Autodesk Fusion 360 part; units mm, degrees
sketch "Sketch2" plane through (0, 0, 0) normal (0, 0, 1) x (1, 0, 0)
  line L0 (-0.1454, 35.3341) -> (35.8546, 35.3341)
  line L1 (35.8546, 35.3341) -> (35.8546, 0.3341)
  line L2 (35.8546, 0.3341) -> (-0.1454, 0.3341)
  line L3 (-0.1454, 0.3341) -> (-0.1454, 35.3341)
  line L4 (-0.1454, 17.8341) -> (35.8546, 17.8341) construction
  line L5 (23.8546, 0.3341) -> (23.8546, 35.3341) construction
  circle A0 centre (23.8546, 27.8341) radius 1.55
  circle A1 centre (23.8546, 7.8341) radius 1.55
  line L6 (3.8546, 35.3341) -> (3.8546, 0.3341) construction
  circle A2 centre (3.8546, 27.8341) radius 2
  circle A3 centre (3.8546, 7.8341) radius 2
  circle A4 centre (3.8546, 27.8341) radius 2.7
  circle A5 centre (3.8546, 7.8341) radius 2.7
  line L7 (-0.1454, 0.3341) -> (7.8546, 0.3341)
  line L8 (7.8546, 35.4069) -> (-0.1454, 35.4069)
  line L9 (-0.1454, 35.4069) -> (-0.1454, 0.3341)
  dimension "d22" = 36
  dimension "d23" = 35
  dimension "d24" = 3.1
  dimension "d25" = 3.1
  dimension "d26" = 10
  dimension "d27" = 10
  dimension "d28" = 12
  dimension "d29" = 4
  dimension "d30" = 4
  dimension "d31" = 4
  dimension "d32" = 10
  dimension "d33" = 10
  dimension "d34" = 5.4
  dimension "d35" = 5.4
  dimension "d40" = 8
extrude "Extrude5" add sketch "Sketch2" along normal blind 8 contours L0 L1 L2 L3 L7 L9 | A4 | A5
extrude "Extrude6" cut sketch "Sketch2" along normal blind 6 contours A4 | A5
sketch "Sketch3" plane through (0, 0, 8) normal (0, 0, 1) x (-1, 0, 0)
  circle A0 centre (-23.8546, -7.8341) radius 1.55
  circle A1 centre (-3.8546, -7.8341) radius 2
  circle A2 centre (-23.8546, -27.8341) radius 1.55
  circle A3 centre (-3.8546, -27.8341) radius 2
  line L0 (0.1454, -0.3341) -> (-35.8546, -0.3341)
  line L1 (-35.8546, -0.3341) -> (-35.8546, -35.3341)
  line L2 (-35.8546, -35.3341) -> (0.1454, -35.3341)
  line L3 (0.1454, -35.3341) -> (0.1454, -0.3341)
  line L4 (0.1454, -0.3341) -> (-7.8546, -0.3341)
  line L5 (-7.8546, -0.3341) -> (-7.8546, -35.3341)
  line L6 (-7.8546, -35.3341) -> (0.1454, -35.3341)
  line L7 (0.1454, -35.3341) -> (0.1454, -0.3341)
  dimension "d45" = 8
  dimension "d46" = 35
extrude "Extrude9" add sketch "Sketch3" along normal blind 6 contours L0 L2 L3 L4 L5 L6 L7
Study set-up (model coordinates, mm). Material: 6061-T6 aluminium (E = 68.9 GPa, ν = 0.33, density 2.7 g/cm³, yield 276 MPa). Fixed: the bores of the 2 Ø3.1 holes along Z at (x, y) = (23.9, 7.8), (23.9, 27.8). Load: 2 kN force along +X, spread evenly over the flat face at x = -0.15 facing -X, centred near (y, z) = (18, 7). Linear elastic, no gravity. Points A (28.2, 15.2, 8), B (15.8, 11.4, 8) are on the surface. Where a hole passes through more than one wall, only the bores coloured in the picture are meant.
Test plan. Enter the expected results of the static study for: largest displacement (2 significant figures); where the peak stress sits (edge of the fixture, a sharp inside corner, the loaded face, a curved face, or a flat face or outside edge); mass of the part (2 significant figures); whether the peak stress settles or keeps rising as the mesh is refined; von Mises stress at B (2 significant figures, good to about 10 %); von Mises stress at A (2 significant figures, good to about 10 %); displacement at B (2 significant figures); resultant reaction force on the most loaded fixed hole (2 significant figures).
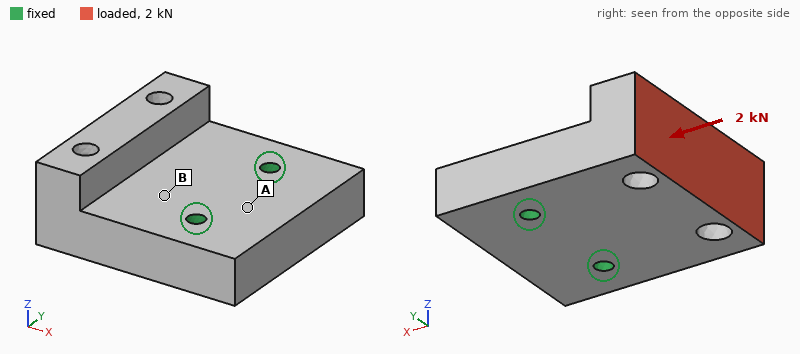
25 µm
edge of the fixture
30 g
keeps rising
22 MPa
5.3 MPa
4.6 µm
1.0 kN
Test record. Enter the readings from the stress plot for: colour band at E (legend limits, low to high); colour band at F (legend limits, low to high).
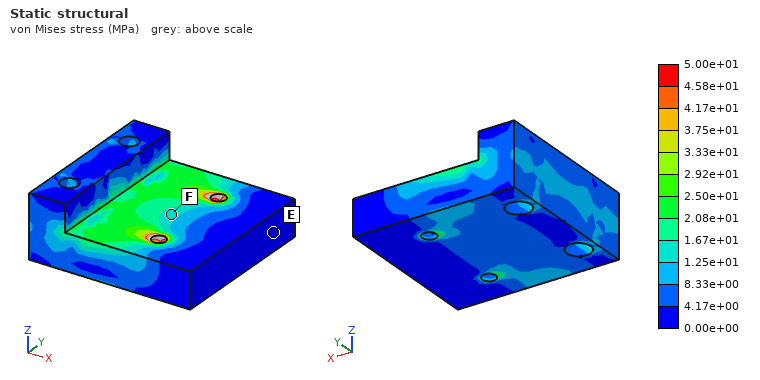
0.00e+00 to 4.17e+00 MPa
1.25e+01 to 1.67e+01 MPa
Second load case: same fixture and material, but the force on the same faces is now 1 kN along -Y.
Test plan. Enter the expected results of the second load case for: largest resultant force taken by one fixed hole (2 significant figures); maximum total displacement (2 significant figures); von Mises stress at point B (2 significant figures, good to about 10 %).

1.2 kN
11 µm
14 MPa
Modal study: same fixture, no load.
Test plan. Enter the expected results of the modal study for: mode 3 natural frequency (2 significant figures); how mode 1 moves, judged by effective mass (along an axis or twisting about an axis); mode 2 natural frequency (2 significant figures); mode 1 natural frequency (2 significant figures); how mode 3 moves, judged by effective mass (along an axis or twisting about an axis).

19 kHz
along Z
14 kHz
7600 Hz
along Y
